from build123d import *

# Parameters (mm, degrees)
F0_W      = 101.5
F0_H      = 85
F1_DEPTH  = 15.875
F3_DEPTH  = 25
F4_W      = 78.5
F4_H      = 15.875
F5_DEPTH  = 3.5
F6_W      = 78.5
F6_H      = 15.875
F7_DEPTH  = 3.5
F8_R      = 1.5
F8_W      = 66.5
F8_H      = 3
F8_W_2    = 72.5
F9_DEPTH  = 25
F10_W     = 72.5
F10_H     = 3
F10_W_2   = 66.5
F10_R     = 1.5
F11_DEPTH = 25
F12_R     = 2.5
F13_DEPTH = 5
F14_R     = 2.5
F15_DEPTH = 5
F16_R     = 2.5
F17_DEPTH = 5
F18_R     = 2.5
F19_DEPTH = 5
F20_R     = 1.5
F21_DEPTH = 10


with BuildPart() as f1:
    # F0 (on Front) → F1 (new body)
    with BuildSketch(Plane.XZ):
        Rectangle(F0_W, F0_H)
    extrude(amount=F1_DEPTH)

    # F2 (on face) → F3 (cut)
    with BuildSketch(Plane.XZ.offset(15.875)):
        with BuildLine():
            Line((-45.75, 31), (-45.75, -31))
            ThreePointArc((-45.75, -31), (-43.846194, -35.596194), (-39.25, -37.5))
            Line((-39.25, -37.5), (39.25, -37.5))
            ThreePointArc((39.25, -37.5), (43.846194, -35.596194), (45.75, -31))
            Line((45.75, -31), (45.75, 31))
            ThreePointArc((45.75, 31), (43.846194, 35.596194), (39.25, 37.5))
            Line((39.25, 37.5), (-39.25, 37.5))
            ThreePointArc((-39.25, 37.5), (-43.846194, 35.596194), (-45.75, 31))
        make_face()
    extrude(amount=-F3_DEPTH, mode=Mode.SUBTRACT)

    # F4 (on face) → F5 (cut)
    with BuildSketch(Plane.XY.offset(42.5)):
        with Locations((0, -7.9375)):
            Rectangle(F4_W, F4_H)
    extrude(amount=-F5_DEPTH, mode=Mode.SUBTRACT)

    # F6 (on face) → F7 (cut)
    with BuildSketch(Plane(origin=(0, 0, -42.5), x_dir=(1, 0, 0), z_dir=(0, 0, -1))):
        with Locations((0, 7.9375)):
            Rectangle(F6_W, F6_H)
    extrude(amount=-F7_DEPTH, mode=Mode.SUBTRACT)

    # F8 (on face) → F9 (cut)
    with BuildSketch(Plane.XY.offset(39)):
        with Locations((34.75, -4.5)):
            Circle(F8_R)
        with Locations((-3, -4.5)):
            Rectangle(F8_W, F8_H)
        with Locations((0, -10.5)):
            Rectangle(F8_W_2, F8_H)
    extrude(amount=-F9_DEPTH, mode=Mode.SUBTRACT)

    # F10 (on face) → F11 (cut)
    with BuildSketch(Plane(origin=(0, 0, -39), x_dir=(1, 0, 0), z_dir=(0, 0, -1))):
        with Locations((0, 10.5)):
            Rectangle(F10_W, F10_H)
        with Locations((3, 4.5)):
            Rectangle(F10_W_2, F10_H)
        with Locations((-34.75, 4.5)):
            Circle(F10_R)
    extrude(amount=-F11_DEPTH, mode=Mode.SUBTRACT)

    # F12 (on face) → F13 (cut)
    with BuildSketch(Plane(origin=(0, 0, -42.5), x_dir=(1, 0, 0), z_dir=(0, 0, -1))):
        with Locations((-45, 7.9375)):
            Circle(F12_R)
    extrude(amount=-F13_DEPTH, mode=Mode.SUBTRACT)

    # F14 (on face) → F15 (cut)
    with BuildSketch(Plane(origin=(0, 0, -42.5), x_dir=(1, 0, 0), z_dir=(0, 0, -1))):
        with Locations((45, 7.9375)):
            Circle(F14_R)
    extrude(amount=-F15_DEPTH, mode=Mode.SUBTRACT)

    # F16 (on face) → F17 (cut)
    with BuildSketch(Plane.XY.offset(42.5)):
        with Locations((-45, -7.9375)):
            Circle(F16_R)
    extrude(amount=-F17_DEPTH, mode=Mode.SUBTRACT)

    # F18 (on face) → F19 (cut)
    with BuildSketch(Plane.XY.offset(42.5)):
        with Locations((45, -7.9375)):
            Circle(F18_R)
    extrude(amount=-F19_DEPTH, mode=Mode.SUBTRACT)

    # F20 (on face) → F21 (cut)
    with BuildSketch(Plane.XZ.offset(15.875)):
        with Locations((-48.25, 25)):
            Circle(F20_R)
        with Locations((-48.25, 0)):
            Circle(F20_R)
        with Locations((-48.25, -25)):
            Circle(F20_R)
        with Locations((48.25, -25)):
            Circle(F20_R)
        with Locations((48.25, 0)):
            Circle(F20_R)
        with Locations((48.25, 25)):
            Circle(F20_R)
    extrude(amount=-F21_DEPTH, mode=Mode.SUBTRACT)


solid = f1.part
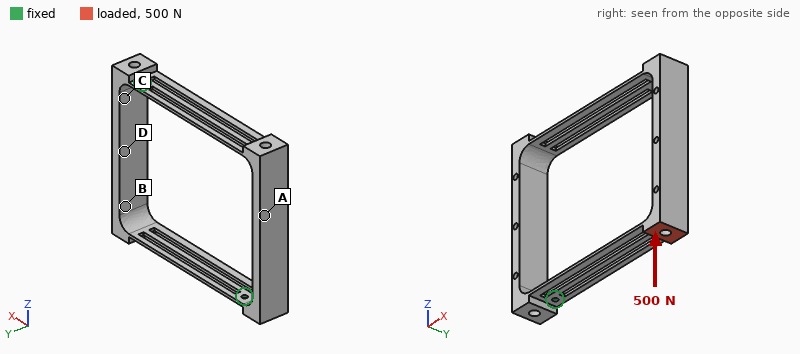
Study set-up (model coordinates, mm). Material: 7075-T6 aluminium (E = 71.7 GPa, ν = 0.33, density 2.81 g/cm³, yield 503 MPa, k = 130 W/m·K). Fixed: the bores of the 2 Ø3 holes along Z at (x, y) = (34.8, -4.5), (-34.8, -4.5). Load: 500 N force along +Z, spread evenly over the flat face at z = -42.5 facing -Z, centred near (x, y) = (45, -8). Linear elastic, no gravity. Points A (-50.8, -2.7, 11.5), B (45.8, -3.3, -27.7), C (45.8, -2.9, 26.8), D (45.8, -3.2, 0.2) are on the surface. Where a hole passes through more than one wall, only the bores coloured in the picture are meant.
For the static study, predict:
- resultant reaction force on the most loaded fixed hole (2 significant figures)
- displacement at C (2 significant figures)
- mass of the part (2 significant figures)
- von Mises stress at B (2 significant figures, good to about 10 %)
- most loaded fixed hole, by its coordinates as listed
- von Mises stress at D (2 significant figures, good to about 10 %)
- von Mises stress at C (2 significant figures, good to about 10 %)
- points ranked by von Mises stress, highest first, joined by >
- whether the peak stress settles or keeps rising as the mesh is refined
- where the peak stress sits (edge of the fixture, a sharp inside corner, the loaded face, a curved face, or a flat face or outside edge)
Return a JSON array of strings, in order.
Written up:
["500 N", "0.18 mm", "50 g", "37 MPa", "(34.8, -4.5)", "56 MPa", "75 MPa", "C > D > B > A", "keeps rising", "edge of the fixture"]
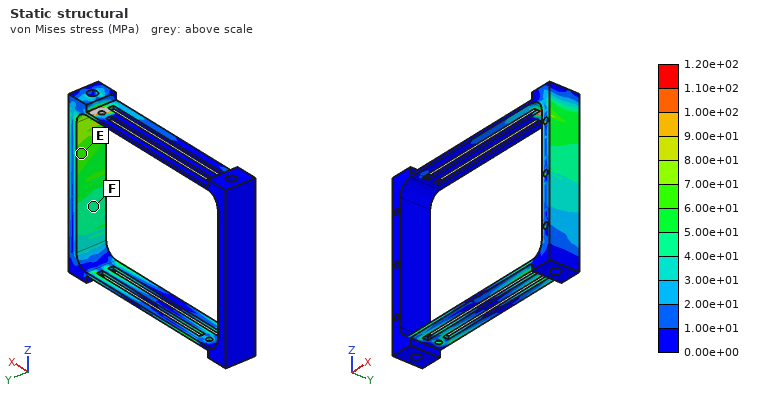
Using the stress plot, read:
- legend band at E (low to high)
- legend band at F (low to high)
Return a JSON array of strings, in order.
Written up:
["6.00e+01 to 7.00e+01 MPa", "4.00e+01 to 5.00e+01 MPa"]
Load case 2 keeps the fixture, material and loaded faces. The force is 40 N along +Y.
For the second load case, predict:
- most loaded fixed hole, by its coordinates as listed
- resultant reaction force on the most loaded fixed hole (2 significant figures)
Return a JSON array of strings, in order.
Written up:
["(-34.8, -4.5)", "23 N"]
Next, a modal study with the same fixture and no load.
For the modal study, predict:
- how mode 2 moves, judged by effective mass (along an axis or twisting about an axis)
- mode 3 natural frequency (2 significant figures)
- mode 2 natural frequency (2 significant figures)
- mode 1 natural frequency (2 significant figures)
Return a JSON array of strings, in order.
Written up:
["along Y", "1200 Hz", "360 Hz", "330 Hz"]
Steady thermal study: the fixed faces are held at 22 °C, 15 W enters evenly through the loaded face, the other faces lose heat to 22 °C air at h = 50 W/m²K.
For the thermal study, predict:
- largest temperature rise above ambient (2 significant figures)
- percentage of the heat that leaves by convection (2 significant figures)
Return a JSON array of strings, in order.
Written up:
["66 K", "70 %"]
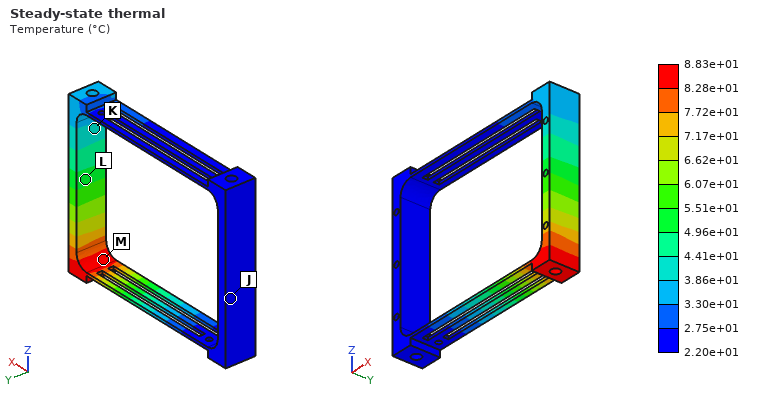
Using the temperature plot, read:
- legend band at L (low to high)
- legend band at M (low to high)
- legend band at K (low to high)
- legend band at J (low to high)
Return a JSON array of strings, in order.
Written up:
["4.96e+01 to 5.51e+01 °C", "8.28e+01 to 8.83e+01 °C", "3.86e+01 to 4.41e+01 °C", "2.20e+01 to 2.75e+01 °C"]
